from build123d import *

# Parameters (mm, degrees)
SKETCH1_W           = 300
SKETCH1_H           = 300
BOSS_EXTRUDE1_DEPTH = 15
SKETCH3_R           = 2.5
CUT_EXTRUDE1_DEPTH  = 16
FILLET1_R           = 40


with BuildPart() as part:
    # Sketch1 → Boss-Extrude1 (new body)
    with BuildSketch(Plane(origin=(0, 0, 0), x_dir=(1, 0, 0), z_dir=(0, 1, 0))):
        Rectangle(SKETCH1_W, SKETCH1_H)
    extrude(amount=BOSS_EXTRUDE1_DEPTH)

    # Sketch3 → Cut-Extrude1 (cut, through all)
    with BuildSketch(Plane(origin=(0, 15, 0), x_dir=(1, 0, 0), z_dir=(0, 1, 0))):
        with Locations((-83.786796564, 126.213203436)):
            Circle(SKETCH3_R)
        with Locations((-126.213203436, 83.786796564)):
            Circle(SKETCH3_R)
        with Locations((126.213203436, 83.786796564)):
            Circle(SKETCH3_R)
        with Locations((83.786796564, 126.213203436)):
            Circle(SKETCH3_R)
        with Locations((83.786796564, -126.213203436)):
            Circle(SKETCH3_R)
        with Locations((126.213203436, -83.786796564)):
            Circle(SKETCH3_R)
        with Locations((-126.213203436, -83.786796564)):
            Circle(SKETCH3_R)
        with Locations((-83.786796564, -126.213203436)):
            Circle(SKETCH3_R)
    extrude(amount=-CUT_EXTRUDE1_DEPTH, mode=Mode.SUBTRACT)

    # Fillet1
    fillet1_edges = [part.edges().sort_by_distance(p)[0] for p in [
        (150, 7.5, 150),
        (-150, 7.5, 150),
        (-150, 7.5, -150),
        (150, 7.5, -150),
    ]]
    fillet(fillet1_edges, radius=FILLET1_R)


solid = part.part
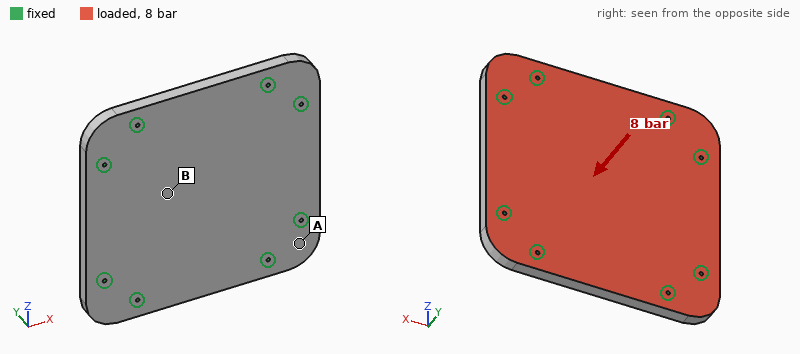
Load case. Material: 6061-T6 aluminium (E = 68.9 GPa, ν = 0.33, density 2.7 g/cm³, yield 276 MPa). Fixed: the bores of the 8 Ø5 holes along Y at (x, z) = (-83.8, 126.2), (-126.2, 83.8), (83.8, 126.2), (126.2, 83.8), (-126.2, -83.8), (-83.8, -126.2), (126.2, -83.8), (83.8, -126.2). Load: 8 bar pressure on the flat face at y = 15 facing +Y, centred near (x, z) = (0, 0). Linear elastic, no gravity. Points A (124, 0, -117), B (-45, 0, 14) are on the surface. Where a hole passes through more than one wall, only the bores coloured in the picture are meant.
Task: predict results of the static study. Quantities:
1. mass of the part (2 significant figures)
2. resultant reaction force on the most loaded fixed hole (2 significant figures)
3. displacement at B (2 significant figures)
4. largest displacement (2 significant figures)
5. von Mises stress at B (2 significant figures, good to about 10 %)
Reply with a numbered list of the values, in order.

1. 3.6 kg
2. 8.9 kN
3. 0.49 mm
4. 0.55 mm
5. 48 MPa
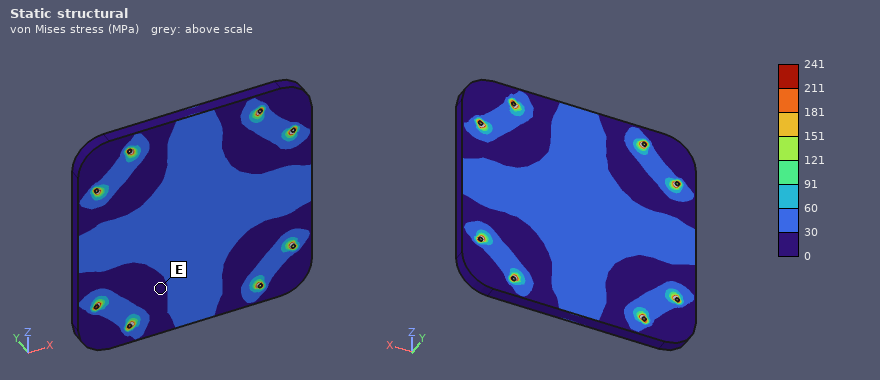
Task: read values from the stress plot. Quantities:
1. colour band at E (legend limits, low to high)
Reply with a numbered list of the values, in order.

1. 0 to 30 MPa
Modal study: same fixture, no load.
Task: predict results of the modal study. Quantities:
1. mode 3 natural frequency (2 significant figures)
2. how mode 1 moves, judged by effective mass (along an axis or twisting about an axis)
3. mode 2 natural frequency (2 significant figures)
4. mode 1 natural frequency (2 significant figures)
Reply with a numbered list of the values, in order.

1. 2200 Hz
2. along Y
3. 2200 Hz
4. 1200 Hz
